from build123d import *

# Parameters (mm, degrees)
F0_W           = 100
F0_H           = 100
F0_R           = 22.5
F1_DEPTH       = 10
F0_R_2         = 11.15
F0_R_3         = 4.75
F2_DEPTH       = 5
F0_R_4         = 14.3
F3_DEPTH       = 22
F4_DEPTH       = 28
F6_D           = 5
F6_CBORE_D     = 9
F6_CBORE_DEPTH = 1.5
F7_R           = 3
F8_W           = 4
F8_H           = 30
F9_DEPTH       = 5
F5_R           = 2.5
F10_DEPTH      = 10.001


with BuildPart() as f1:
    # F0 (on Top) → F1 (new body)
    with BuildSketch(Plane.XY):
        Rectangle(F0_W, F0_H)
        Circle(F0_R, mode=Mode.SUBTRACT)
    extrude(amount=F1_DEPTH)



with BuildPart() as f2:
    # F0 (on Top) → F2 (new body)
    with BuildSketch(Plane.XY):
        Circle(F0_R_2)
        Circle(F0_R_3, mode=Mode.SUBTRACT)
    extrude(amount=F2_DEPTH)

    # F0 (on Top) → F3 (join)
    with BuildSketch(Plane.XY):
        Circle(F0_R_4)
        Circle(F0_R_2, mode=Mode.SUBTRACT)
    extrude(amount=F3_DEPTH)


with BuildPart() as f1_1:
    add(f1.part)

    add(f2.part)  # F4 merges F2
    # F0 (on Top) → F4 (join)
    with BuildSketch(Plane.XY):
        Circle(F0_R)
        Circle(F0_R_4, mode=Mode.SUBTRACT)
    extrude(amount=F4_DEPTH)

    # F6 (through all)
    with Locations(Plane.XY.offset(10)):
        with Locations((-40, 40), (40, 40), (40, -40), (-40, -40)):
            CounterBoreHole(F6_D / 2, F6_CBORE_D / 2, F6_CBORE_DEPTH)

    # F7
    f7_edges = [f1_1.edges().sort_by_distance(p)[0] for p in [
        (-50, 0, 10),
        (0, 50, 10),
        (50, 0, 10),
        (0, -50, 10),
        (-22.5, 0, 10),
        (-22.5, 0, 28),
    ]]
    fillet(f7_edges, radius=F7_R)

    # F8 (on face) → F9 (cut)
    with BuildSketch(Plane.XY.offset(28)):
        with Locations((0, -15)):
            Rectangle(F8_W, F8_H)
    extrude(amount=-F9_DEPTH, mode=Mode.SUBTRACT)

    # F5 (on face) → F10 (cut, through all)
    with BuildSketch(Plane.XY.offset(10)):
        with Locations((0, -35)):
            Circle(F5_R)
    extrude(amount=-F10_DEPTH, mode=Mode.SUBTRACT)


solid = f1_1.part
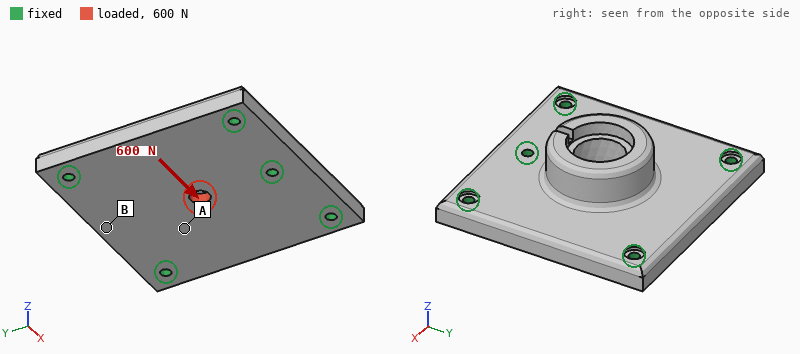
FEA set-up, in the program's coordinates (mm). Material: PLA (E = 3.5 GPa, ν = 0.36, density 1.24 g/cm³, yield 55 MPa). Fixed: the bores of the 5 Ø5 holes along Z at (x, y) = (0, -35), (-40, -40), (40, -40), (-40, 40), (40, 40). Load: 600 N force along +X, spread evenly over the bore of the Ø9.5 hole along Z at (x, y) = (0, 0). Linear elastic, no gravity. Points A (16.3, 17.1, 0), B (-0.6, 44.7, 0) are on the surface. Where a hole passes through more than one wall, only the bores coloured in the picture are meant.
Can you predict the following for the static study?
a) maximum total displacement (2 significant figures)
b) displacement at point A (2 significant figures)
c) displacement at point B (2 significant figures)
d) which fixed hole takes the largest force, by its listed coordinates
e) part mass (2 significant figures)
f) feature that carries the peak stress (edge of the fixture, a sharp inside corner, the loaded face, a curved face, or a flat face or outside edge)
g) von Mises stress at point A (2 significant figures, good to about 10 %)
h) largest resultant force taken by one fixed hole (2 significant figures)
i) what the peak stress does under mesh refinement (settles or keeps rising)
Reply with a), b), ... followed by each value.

a) 23 µm
b) 9.5 µm
c) 3.6 µm
d) (0, -35)
e) 140 g
f) a sharp inside corner
g) 0.96 MPa
h) 170 N
i) keeps rising
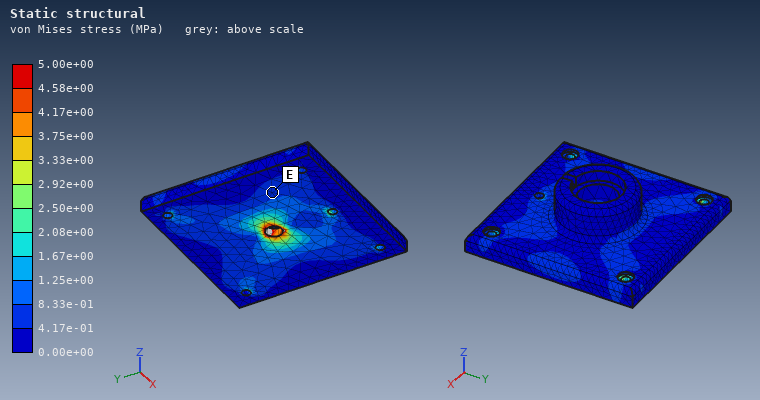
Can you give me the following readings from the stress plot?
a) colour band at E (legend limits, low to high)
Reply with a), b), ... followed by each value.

a) 4.17e-01 to 8.33e-01 MPa
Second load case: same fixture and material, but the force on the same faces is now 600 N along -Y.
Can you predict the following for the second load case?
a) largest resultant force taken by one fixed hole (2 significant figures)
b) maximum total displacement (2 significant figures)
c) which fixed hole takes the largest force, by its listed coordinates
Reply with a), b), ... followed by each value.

a) 230 N
b) 21 µm
c) (0, -35)
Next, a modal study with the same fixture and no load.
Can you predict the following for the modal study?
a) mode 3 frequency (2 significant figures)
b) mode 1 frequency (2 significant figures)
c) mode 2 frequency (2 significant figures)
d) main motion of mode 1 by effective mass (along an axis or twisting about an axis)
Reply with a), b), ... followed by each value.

a) 2800 Hz
b) 1700 Hz
c) 2300 Hz
d) along Z
